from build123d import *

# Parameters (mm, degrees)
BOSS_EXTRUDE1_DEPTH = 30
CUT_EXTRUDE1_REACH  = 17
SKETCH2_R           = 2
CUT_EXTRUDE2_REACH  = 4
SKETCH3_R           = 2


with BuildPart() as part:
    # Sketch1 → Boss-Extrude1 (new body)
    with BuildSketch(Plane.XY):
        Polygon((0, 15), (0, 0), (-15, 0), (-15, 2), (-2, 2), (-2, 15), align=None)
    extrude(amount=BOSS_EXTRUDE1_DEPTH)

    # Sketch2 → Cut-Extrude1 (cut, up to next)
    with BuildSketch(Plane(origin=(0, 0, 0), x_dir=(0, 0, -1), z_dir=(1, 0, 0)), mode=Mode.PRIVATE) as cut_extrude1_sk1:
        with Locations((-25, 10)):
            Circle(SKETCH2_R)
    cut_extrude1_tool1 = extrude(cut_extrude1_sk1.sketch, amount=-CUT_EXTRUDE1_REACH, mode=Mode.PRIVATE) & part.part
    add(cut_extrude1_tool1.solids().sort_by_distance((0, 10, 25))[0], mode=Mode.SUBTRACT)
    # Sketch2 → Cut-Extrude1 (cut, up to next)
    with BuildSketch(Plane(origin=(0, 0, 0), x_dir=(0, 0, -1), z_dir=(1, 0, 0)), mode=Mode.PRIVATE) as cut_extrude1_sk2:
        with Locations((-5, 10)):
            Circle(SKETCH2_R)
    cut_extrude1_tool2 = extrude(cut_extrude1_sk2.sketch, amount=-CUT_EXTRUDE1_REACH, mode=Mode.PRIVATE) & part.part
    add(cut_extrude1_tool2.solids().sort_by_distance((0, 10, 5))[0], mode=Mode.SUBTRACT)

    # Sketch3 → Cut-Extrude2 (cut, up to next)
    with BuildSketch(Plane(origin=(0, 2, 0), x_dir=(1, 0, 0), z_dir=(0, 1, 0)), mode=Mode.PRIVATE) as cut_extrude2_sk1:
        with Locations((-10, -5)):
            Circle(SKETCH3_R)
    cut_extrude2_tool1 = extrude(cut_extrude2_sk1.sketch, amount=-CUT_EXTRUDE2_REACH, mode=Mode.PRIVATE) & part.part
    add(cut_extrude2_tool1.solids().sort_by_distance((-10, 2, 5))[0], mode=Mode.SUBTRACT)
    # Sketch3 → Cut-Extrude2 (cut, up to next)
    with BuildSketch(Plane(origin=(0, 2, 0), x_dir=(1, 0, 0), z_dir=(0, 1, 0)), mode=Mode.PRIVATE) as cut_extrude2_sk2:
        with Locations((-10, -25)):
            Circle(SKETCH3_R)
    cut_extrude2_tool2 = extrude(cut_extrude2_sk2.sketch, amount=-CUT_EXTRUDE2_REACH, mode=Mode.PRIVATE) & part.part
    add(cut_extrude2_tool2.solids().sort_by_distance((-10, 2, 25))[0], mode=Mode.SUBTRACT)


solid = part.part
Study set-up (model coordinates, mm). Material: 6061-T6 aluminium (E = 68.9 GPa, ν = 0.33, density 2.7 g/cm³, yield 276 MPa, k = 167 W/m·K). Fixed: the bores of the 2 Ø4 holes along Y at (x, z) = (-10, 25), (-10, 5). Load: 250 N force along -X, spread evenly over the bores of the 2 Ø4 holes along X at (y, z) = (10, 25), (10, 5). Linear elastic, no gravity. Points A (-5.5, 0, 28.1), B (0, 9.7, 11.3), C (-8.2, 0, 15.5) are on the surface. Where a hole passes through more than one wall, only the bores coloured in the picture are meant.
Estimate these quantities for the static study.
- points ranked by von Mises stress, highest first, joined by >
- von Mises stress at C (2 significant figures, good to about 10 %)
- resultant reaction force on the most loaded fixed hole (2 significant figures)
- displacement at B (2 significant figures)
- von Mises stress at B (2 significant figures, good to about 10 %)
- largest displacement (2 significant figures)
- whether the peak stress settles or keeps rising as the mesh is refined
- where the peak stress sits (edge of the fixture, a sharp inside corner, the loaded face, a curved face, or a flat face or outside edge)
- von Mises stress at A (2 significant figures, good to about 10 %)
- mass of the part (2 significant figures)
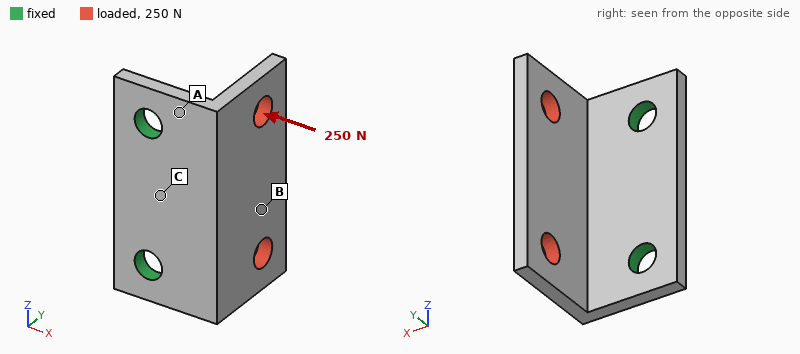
A > C > B
52 MPa
130 N
0.15 mm
22 MPa
0.26 mm
keeps rising
edge of the fixture
110 MPa
4.3 g
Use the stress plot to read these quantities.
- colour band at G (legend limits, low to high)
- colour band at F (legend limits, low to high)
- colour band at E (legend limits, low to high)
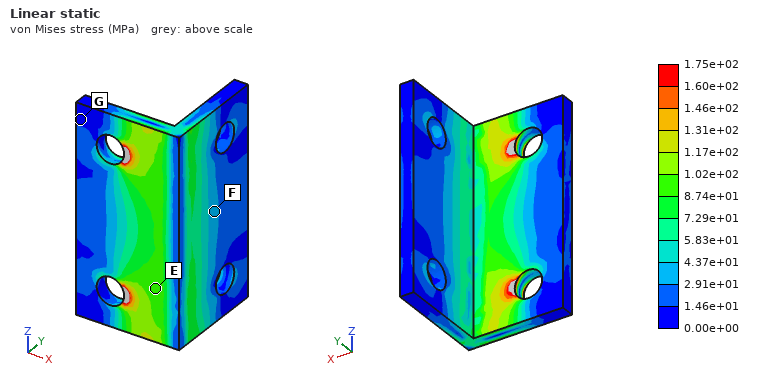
0.00e+00 to 1.46e+01 MPa
2.91e+01 to 4.37e+01 MPa
8.74e+01 to 1.02e+02 MPa
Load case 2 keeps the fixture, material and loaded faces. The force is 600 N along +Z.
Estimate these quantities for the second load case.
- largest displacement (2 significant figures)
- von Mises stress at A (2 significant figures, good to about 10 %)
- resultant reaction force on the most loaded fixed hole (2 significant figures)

0.11 mm
81 MPa
450 N
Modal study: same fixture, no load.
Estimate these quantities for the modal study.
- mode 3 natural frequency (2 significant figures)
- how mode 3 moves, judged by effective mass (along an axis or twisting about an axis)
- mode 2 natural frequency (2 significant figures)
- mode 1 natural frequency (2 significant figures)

13 kHz
along Y
8100 Hz
4500 Hz
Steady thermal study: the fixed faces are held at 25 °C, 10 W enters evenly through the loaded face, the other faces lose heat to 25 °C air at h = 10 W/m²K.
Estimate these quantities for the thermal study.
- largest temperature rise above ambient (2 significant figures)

21 K
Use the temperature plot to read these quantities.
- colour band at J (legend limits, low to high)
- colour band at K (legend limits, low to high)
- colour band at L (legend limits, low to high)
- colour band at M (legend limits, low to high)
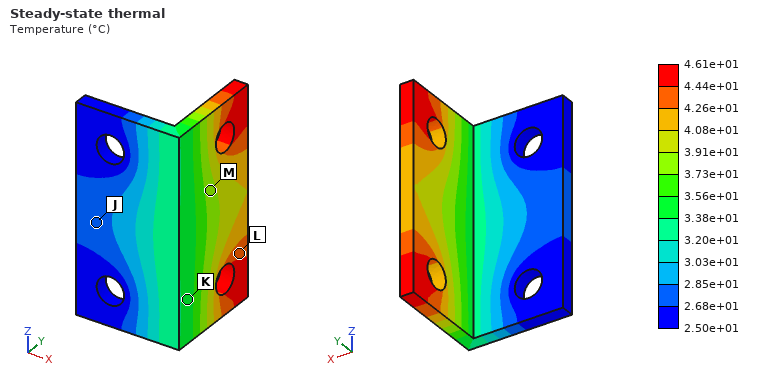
2.68e+01 to 2.85e+01 °C
3.38e+01 to 3.56e+01 °C
4.26e+01 to 4.44e+01 °C
3.73e+01 to 3.91e+01 °C
